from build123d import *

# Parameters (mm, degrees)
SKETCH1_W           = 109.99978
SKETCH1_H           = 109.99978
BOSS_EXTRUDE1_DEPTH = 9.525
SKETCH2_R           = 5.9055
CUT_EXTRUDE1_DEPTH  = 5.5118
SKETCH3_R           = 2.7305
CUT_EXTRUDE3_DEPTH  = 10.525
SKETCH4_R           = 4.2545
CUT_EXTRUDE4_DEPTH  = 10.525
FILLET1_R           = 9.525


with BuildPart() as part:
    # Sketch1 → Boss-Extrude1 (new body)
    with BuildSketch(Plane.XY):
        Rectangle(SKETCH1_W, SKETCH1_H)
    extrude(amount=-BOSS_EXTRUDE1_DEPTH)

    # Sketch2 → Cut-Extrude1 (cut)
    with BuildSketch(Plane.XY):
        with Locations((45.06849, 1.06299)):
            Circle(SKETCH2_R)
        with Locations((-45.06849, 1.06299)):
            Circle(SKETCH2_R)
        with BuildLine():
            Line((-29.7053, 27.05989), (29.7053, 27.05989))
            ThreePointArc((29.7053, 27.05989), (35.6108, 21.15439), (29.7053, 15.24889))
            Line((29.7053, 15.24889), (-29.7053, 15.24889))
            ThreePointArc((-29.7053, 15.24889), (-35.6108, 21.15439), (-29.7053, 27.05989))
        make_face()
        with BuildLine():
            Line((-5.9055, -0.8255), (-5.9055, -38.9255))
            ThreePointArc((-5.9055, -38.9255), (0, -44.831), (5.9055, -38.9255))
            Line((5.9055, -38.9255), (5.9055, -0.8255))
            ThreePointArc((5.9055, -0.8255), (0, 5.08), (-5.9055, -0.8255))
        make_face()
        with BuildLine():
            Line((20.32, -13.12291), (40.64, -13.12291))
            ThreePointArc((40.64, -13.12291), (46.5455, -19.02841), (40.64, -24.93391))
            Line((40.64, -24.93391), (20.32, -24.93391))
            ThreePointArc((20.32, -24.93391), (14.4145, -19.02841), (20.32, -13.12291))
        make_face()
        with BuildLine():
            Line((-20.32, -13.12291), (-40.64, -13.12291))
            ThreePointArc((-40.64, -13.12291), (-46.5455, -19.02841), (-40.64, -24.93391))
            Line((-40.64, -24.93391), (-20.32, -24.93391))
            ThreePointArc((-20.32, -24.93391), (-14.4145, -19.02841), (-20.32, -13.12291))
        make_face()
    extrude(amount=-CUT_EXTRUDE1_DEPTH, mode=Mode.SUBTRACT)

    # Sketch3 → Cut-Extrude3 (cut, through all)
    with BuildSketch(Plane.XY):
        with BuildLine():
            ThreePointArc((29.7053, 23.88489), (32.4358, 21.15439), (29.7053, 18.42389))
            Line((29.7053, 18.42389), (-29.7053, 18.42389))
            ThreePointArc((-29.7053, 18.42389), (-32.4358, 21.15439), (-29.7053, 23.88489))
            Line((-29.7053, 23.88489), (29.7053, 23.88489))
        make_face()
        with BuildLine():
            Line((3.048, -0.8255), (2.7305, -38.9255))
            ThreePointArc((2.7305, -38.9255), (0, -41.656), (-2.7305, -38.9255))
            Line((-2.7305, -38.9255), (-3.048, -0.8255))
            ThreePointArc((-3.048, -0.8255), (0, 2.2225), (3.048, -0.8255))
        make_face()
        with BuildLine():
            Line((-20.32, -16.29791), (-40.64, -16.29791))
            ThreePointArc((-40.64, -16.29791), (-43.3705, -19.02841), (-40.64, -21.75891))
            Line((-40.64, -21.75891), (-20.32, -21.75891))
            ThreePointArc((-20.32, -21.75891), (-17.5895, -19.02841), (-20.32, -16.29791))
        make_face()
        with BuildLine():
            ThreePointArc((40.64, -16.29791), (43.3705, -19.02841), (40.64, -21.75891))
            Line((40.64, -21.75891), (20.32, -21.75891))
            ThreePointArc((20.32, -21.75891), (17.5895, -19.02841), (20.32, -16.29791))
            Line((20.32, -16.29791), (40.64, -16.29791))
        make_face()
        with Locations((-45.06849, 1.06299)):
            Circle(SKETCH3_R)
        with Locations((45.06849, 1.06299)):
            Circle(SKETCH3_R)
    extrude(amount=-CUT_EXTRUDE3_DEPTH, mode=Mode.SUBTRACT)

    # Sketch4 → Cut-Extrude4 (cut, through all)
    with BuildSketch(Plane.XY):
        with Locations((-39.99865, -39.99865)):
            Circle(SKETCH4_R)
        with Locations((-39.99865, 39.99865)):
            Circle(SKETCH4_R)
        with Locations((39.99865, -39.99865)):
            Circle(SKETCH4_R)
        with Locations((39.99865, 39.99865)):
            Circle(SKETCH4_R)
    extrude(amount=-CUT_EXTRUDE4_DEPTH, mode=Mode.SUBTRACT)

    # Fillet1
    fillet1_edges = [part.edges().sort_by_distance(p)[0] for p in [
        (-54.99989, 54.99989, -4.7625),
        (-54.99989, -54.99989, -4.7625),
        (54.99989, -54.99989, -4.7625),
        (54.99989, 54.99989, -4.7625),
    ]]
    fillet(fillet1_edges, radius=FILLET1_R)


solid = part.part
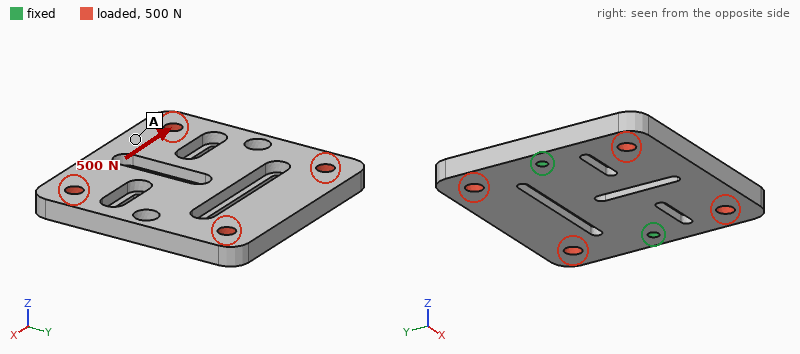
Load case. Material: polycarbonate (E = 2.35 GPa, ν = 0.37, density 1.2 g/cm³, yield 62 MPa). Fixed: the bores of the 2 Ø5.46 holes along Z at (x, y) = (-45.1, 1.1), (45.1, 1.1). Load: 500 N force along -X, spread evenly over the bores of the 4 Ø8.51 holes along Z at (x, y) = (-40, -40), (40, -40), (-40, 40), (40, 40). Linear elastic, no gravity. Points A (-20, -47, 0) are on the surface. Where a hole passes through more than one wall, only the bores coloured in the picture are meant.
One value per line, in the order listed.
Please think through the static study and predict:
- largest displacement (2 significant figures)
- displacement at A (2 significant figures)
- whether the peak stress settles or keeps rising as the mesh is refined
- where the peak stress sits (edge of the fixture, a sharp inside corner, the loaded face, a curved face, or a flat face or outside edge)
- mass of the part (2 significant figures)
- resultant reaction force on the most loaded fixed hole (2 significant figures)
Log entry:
65 µm
57 µm
keeps rising
edge of the fixture
120 g
250 N
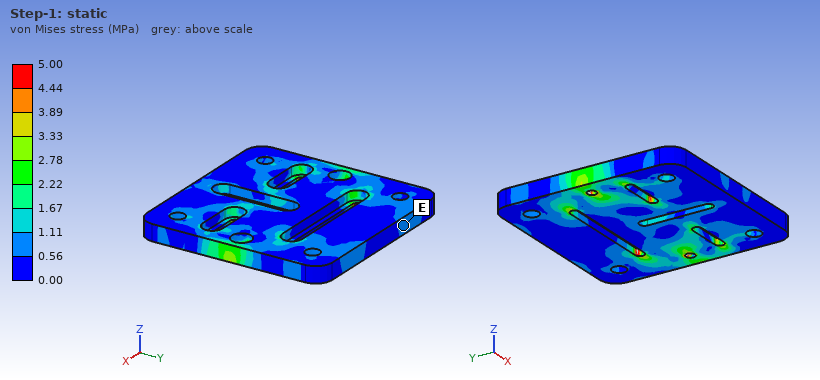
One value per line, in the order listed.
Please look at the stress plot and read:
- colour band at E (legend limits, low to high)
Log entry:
0.56 to 1.11 MPa
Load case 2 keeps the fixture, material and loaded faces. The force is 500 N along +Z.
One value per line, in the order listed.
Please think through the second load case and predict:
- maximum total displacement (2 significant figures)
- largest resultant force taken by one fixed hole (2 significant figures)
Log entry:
1.2 mm
270 N
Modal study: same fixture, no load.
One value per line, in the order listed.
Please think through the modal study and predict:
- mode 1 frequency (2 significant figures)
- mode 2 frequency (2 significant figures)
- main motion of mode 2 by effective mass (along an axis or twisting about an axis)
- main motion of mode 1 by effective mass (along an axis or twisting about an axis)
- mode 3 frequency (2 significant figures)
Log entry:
240 Hz
450 Hz
along Z
twisting about X
680 Hz
